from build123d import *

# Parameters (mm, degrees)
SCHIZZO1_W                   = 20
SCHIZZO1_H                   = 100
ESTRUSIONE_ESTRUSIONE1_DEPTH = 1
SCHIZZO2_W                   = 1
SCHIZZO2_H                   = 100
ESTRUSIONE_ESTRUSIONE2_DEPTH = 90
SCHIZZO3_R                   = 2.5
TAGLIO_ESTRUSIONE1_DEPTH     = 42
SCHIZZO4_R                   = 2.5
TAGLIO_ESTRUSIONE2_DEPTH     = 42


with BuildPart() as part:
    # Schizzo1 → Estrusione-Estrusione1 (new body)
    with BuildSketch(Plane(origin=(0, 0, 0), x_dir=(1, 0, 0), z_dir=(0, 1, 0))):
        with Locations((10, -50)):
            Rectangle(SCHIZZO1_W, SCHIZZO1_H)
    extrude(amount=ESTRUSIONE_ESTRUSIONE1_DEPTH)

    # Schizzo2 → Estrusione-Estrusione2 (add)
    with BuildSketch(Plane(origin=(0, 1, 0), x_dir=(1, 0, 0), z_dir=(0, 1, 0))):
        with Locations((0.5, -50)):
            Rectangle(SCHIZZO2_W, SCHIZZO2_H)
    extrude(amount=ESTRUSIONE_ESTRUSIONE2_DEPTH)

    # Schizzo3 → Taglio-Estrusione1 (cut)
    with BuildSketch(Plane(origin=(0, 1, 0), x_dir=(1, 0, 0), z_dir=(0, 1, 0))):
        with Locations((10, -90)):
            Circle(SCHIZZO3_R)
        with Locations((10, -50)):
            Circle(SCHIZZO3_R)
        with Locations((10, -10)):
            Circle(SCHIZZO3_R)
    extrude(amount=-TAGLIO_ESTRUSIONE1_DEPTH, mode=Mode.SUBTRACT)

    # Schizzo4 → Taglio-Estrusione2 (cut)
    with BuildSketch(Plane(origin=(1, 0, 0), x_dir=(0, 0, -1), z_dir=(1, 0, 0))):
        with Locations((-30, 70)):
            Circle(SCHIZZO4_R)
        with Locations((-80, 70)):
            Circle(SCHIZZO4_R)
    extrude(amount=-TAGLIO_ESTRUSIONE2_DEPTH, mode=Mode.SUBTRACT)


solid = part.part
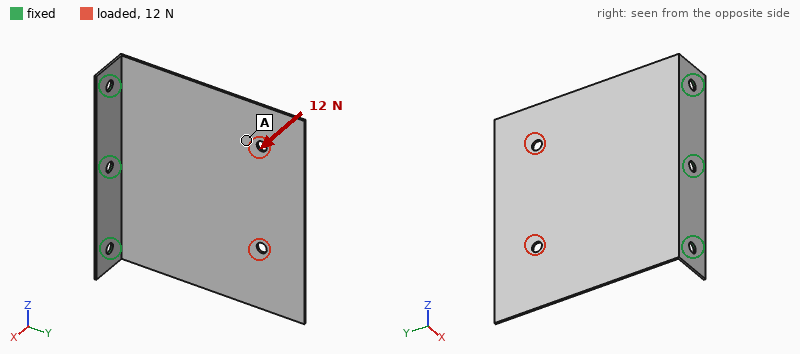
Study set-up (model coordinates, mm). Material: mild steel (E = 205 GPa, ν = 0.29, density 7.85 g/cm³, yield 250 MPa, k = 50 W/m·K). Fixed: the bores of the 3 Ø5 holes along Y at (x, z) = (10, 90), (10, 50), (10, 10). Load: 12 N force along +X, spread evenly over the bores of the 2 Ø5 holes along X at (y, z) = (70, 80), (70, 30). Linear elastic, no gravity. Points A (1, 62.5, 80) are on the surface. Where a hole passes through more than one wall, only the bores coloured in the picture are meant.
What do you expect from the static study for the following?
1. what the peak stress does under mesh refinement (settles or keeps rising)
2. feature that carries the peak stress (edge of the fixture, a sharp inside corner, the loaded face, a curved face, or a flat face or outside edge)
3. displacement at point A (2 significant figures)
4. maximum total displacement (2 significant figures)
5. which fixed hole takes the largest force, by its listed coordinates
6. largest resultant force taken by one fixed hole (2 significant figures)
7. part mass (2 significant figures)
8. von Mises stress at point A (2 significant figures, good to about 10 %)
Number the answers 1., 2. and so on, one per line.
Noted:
1. keeps rising
2. edge of the fixture
3. 0.89 mm
4. 1.5 mm
5. (10, 50)
6. 12 N
7. 86 g
8. 8.7 MPa
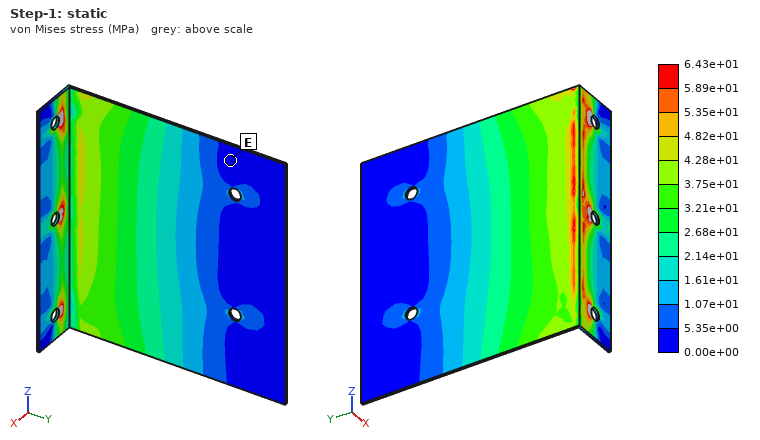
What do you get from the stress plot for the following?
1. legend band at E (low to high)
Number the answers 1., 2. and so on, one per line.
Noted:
1. 0.00e+00 to 5.35e+00 MPa
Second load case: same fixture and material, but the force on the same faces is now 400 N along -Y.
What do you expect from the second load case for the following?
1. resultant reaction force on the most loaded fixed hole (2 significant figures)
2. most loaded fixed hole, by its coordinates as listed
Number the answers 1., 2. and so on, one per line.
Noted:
1. 160 N
2. (10, 90)
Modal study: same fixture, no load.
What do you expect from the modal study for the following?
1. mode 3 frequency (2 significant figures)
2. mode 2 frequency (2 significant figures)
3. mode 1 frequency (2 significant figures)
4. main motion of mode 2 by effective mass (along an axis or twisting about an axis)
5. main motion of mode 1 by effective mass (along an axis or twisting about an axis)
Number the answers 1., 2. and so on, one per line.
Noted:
1. 550 Hz
2. 220 Hz
3. 88 Hz
4. twisting about Y
5. along X
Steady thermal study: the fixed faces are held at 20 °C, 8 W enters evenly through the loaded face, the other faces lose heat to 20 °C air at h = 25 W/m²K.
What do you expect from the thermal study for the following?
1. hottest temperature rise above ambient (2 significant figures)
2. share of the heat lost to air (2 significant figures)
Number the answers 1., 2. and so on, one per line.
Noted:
1. 49 K
2. 91 %
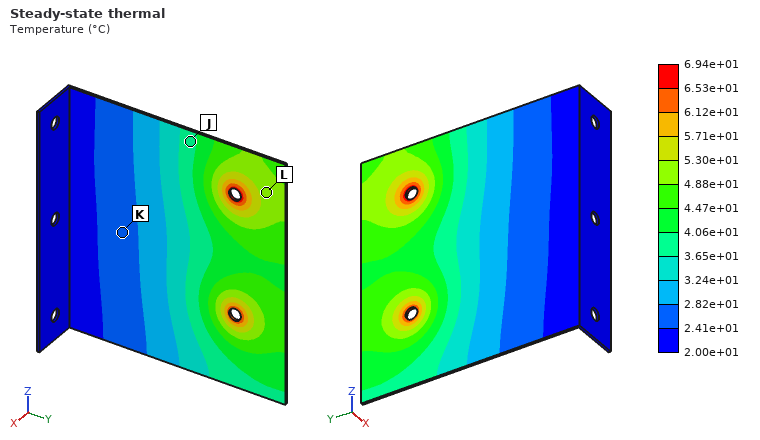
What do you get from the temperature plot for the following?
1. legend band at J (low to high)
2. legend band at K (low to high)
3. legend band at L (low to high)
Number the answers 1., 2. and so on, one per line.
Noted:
1. 3.65e+01 to 4.06e+01 °C
2. 2.41e+01 to 2.82e+01 °C
3. 4.88e+01 to 5.30e+01 °C
